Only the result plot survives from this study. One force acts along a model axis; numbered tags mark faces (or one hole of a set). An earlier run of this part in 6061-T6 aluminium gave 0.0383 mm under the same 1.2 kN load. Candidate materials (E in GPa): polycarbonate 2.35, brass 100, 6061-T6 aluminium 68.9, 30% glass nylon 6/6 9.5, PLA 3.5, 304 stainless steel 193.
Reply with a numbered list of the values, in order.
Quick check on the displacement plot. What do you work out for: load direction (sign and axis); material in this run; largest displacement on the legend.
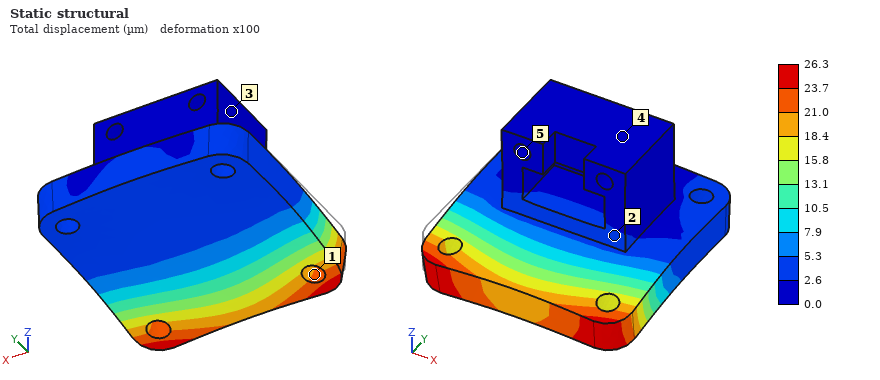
1. -Z
2. brass
3. 26.3 µm
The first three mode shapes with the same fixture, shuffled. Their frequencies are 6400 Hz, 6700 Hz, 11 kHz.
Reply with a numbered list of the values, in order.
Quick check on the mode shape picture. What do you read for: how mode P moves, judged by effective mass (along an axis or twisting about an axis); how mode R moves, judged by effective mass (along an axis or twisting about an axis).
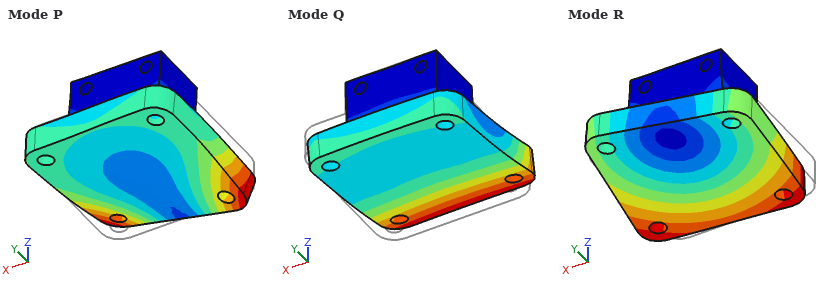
1. along X
2. along X
